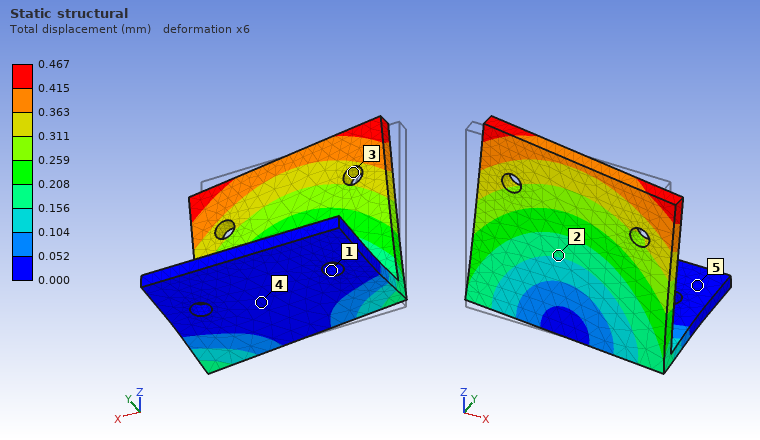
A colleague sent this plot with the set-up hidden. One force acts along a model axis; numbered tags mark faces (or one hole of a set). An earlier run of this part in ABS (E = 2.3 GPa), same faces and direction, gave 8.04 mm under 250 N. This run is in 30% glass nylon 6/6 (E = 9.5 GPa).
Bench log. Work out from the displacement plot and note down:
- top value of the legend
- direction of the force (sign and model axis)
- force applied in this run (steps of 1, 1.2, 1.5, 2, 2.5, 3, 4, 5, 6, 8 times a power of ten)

0.467 mm
+X
60 N
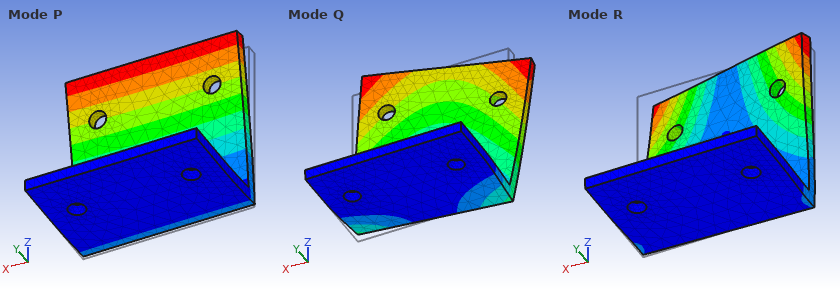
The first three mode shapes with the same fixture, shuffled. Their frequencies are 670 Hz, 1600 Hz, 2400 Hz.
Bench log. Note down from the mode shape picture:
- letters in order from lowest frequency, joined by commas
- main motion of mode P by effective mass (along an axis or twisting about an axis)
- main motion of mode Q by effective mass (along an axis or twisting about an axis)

P, Q, R
along Y
along X
